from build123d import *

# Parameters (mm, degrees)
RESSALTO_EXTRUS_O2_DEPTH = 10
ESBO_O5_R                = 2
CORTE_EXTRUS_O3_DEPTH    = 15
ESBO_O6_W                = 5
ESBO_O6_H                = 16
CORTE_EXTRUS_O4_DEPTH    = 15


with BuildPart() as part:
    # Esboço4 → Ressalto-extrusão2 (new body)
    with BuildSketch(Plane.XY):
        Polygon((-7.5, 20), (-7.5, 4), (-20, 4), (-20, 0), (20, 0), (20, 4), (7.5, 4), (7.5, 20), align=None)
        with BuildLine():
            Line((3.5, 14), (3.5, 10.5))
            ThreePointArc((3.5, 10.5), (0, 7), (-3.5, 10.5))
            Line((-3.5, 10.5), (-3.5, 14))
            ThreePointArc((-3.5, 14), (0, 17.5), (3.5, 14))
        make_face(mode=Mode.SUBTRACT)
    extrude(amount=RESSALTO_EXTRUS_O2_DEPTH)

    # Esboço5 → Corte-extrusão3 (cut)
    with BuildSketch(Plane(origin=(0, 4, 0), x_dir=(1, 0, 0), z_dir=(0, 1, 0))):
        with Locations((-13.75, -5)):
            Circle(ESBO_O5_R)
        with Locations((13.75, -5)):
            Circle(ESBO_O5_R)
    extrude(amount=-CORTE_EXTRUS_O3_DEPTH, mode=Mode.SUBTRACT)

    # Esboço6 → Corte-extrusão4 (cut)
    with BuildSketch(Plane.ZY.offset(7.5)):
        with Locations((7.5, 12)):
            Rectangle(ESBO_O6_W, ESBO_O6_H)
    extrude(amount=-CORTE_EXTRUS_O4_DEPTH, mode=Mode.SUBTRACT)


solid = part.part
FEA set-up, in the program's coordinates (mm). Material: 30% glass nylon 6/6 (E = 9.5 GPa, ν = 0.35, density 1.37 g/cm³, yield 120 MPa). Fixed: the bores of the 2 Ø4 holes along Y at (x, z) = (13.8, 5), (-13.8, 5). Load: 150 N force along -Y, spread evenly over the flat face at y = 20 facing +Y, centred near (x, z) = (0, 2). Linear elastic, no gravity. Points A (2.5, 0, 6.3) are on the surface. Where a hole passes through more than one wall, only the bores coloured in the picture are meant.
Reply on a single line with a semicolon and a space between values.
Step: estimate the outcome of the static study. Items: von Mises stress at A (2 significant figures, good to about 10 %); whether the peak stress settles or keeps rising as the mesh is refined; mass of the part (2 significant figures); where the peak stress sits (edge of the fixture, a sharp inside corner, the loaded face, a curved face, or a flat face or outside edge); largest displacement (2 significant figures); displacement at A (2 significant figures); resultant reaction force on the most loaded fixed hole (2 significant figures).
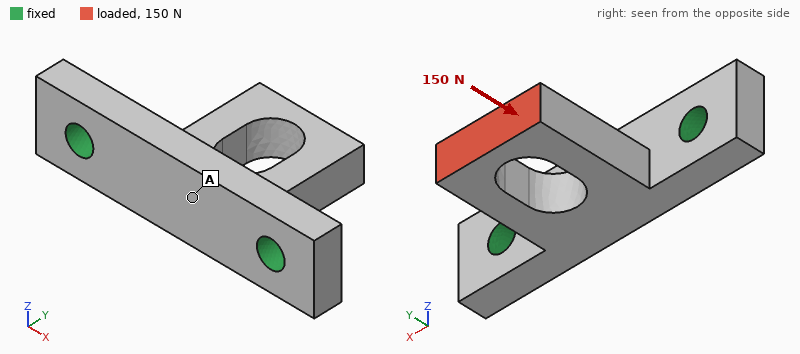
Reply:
2.6 MPa; keeps rising; 3.3 g; edge of the fixture; 41 µm; 9.1 µm; 78 N
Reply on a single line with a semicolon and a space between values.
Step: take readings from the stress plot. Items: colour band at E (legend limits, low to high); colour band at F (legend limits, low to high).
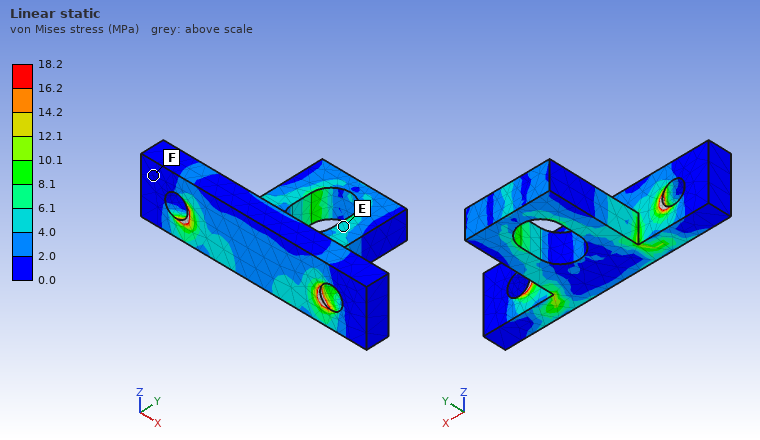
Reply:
4.0 to 6.1 MPa; 0.0 to 2.0 MPa
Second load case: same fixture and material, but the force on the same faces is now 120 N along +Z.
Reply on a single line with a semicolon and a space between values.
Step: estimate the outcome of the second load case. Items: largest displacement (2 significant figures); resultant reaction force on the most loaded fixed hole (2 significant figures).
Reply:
0.45 mm; 61 N
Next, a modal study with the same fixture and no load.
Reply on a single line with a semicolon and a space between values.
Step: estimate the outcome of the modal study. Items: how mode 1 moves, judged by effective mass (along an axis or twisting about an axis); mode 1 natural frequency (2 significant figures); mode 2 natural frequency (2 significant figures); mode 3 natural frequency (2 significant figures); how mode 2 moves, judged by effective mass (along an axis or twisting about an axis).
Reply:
along Z; 4100 Hz; 8500 Hz; 11 kHz; along X
